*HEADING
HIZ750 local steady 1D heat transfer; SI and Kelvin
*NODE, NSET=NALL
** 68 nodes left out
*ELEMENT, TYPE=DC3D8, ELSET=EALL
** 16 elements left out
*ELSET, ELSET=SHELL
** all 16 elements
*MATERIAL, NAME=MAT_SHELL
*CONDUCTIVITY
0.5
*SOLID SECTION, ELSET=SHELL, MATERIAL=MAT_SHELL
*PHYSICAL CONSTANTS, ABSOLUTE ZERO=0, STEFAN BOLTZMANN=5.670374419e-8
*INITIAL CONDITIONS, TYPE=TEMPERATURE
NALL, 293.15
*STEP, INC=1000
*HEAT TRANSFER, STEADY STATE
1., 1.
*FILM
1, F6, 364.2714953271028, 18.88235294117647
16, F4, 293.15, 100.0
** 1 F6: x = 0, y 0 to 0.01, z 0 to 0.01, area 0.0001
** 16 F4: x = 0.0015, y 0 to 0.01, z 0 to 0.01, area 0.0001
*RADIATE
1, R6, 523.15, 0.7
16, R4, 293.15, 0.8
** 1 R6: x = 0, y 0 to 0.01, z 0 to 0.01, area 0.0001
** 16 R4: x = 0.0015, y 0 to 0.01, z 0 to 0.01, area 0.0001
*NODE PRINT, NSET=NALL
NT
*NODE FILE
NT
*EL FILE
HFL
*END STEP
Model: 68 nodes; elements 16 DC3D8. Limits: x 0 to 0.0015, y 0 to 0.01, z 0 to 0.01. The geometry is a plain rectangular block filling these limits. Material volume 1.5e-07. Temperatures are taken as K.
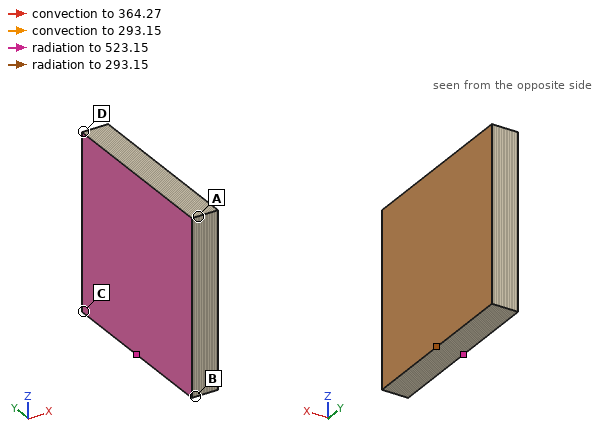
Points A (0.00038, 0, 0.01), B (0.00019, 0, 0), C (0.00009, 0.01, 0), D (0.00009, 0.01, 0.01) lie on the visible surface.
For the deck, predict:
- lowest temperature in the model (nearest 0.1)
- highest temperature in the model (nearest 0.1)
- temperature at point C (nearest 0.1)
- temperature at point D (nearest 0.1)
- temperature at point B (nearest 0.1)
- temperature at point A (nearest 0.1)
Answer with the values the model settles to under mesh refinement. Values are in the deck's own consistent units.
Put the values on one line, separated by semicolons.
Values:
322.6 K; 331.9 K; 331.3 K; 331.3 K; 330.8 K; 329.6 K
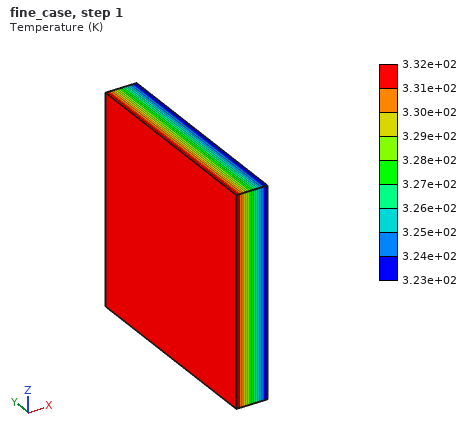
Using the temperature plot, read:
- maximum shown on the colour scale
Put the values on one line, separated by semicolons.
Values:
3.32e+02 K
